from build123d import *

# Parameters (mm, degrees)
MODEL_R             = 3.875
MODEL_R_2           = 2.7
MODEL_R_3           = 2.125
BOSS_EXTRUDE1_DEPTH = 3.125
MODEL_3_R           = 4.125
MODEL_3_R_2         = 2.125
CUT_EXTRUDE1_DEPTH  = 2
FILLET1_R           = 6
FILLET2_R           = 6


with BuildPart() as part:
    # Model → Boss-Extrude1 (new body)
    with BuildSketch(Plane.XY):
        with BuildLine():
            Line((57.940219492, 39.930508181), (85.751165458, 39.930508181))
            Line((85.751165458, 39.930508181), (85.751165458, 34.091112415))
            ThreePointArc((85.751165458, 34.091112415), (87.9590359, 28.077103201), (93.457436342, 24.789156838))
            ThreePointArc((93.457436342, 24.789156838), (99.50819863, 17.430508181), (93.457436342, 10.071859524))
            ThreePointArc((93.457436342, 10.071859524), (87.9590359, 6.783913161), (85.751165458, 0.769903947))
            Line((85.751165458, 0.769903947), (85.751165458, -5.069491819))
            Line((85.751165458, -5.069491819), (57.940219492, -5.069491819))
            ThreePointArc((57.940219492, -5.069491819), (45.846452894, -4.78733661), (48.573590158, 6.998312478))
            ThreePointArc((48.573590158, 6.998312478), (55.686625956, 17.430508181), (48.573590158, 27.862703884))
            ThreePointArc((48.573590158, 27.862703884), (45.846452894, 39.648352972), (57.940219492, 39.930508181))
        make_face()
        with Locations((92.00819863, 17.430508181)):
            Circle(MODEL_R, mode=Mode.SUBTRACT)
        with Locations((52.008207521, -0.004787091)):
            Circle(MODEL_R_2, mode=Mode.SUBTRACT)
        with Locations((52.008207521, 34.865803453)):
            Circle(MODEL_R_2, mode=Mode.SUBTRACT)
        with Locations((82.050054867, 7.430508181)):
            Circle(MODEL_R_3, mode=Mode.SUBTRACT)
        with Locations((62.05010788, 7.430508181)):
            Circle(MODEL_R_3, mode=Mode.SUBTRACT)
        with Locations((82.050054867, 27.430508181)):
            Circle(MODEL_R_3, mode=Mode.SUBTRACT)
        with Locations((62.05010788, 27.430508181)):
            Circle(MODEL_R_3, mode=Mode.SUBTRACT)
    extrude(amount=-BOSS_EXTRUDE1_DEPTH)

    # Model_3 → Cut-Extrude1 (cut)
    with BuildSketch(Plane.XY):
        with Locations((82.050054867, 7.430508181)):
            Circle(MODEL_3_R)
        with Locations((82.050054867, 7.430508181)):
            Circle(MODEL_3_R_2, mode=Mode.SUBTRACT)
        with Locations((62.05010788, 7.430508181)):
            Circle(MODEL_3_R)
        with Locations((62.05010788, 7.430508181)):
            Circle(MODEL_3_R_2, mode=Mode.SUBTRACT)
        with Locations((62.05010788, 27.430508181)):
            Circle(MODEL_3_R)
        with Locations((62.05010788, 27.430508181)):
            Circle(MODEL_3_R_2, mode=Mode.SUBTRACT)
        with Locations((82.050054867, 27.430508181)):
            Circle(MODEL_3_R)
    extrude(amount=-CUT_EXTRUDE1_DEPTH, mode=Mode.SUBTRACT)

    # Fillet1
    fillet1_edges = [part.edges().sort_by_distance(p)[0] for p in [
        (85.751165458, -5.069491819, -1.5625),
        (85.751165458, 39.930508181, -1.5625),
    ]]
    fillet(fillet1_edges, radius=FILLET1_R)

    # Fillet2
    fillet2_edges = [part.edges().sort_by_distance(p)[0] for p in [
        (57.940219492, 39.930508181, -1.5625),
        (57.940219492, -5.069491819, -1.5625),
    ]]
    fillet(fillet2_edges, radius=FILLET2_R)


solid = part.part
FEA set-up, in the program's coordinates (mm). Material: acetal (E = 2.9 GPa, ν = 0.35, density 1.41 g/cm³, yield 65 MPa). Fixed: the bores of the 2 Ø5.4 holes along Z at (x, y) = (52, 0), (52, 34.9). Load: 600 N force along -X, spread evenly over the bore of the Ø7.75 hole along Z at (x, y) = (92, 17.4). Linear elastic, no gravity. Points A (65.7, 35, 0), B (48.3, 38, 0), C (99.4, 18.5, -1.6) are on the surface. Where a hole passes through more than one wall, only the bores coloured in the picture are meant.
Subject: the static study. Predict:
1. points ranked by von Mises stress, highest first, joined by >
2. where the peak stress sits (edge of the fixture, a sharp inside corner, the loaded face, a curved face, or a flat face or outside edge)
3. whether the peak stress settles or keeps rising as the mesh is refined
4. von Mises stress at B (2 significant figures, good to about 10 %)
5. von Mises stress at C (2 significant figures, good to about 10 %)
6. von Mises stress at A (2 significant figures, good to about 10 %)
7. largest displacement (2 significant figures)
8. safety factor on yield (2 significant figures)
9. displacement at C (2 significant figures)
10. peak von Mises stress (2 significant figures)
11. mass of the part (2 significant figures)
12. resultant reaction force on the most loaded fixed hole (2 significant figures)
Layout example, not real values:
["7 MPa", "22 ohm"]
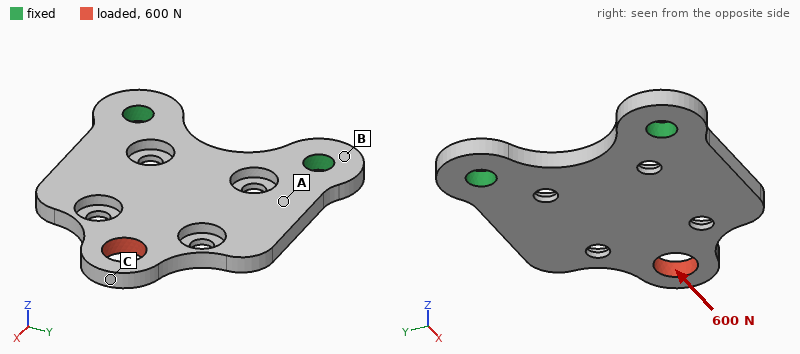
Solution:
["C > A > B", "a curved face", "settles", "2.3 MPa", "14 MPa", "7.0 MPa", "0.38 mm", "1.9", "0.37 mm", "35 MPa", "7.2 g", "320 N"]
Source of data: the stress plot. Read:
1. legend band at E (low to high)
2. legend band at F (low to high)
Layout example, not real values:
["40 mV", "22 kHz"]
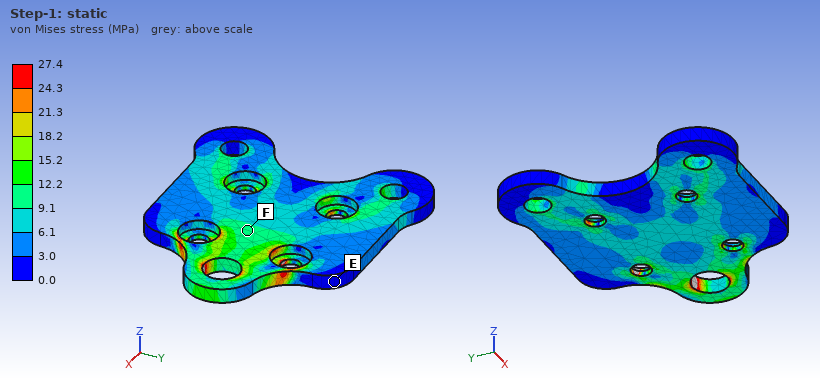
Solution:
["0.0 to 3.0 MPa", "9.1 to 12.2 MPa"]
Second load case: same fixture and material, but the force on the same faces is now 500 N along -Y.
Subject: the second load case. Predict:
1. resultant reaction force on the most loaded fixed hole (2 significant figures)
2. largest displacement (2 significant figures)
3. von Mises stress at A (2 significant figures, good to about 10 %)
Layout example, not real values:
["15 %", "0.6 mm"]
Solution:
["580 N", "0.62 mm", "12 MPa"]
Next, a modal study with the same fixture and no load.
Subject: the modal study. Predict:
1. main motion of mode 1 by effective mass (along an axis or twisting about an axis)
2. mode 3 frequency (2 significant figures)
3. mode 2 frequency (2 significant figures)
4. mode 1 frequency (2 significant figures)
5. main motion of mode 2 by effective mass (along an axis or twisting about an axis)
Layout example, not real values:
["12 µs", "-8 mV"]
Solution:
["along Z", "2000 Hz", "1300 Hz", "460 Hz", "twisting about X"]
